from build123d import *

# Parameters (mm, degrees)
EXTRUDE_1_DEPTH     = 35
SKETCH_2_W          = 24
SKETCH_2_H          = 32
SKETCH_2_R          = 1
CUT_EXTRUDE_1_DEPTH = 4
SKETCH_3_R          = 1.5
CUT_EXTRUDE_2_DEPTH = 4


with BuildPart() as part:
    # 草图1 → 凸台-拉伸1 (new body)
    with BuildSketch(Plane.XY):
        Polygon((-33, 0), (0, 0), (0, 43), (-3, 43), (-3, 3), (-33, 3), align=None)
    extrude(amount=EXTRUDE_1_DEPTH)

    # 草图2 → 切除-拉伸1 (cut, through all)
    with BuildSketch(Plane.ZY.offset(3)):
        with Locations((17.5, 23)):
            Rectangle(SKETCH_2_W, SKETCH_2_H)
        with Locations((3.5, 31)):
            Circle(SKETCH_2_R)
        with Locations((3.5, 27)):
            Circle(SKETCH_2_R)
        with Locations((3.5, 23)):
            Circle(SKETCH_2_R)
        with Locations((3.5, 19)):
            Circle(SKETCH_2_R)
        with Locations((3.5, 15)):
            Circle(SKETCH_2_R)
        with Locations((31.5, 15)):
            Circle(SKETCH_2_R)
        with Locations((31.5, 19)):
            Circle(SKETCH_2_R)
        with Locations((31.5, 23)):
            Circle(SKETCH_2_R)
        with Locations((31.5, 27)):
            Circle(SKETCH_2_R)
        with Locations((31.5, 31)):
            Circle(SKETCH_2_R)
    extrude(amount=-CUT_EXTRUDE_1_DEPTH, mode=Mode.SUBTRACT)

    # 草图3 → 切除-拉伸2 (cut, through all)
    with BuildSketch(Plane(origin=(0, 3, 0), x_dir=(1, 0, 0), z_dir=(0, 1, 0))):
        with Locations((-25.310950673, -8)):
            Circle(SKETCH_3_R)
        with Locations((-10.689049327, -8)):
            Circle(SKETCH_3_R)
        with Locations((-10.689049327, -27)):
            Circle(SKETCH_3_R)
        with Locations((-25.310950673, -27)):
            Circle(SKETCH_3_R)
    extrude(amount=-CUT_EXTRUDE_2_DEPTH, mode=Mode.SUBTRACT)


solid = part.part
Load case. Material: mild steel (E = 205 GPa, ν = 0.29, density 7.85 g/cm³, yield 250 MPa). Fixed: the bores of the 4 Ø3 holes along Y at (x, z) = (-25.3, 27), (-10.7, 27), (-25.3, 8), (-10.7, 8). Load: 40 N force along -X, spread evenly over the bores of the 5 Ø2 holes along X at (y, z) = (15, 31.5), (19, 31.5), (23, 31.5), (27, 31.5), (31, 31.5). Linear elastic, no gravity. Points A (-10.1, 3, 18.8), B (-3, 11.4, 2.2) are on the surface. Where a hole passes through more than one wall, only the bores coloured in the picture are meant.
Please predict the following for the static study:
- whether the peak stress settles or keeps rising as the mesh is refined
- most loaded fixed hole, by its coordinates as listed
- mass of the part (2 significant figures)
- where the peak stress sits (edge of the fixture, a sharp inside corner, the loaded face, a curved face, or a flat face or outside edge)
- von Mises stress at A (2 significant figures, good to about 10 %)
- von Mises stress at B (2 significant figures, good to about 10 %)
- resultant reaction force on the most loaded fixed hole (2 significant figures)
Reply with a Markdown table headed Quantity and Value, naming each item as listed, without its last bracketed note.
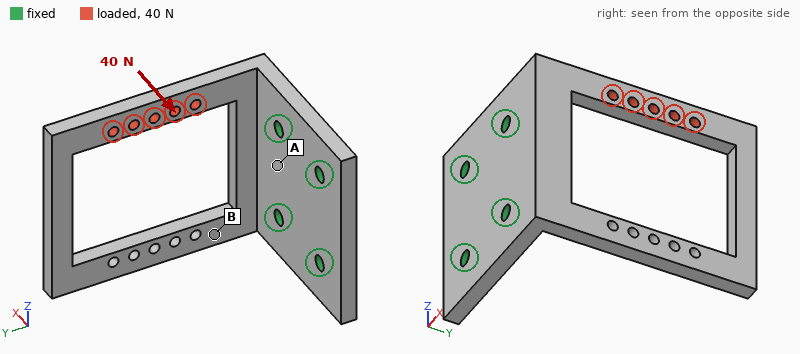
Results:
| Quantity | Value |
|---|---|
| whether the peak stress settles or keeps rising as the mesh is refined | keeps rising |
| most loaded fixed hole, by its coordinates as listed | (-10.7, 27) |
| mass of the part | 41 g |
| where the peak stress sits | a sharp inside corner |
| von Mises stress at A | 8.6 MPa |
| von Mises stress at B | 21 MPa |
| resultant reaction force on the most loaded fixed hole | 37 N |
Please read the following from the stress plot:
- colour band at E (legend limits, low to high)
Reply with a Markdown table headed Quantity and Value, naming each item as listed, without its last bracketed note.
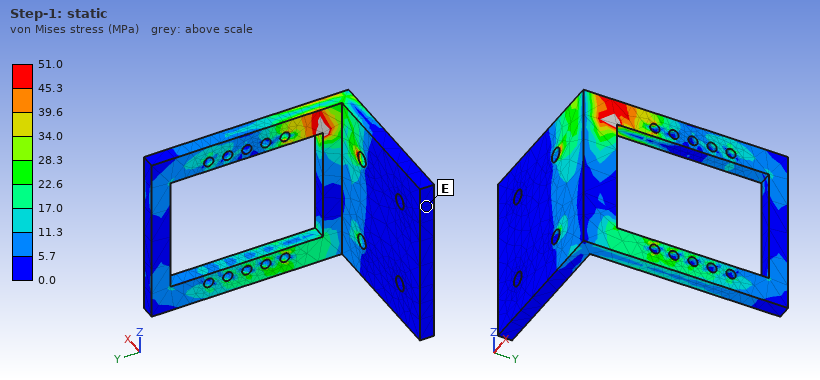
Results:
| Quantity | Value |
|---|---|
| colour band at E | 0.0 to 5.7 MPa |
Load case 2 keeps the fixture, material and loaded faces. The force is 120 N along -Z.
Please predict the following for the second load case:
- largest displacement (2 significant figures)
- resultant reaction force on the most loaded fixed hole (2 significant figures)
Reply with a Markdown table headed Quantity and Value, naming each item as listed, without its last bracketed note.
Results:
| Quantity | Value |
|---|---|
| largest displacement | 40 µm |
| resultant reaction force on the most loaded fixed hole | 140 N |
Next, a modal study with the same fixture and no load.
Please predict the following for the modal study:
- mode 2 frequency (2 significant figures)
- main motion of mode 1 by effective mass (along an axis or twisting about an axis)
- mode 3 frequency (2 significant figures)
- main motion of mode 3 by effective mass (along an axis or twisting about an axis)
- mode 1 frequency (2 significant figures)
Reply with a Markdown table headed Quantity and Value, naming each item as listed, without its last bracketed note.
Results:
| Quantity | Value |
|---|---|
| mode 2 frequency | 2300 Hz |
| main motion of mode 1 by effective mass | along X |
| mode 3 frequency | 2700 Hz |
| main motion of mode 3 by effective mass | along Z |
| mode 1 frequency | 990 Hz |
